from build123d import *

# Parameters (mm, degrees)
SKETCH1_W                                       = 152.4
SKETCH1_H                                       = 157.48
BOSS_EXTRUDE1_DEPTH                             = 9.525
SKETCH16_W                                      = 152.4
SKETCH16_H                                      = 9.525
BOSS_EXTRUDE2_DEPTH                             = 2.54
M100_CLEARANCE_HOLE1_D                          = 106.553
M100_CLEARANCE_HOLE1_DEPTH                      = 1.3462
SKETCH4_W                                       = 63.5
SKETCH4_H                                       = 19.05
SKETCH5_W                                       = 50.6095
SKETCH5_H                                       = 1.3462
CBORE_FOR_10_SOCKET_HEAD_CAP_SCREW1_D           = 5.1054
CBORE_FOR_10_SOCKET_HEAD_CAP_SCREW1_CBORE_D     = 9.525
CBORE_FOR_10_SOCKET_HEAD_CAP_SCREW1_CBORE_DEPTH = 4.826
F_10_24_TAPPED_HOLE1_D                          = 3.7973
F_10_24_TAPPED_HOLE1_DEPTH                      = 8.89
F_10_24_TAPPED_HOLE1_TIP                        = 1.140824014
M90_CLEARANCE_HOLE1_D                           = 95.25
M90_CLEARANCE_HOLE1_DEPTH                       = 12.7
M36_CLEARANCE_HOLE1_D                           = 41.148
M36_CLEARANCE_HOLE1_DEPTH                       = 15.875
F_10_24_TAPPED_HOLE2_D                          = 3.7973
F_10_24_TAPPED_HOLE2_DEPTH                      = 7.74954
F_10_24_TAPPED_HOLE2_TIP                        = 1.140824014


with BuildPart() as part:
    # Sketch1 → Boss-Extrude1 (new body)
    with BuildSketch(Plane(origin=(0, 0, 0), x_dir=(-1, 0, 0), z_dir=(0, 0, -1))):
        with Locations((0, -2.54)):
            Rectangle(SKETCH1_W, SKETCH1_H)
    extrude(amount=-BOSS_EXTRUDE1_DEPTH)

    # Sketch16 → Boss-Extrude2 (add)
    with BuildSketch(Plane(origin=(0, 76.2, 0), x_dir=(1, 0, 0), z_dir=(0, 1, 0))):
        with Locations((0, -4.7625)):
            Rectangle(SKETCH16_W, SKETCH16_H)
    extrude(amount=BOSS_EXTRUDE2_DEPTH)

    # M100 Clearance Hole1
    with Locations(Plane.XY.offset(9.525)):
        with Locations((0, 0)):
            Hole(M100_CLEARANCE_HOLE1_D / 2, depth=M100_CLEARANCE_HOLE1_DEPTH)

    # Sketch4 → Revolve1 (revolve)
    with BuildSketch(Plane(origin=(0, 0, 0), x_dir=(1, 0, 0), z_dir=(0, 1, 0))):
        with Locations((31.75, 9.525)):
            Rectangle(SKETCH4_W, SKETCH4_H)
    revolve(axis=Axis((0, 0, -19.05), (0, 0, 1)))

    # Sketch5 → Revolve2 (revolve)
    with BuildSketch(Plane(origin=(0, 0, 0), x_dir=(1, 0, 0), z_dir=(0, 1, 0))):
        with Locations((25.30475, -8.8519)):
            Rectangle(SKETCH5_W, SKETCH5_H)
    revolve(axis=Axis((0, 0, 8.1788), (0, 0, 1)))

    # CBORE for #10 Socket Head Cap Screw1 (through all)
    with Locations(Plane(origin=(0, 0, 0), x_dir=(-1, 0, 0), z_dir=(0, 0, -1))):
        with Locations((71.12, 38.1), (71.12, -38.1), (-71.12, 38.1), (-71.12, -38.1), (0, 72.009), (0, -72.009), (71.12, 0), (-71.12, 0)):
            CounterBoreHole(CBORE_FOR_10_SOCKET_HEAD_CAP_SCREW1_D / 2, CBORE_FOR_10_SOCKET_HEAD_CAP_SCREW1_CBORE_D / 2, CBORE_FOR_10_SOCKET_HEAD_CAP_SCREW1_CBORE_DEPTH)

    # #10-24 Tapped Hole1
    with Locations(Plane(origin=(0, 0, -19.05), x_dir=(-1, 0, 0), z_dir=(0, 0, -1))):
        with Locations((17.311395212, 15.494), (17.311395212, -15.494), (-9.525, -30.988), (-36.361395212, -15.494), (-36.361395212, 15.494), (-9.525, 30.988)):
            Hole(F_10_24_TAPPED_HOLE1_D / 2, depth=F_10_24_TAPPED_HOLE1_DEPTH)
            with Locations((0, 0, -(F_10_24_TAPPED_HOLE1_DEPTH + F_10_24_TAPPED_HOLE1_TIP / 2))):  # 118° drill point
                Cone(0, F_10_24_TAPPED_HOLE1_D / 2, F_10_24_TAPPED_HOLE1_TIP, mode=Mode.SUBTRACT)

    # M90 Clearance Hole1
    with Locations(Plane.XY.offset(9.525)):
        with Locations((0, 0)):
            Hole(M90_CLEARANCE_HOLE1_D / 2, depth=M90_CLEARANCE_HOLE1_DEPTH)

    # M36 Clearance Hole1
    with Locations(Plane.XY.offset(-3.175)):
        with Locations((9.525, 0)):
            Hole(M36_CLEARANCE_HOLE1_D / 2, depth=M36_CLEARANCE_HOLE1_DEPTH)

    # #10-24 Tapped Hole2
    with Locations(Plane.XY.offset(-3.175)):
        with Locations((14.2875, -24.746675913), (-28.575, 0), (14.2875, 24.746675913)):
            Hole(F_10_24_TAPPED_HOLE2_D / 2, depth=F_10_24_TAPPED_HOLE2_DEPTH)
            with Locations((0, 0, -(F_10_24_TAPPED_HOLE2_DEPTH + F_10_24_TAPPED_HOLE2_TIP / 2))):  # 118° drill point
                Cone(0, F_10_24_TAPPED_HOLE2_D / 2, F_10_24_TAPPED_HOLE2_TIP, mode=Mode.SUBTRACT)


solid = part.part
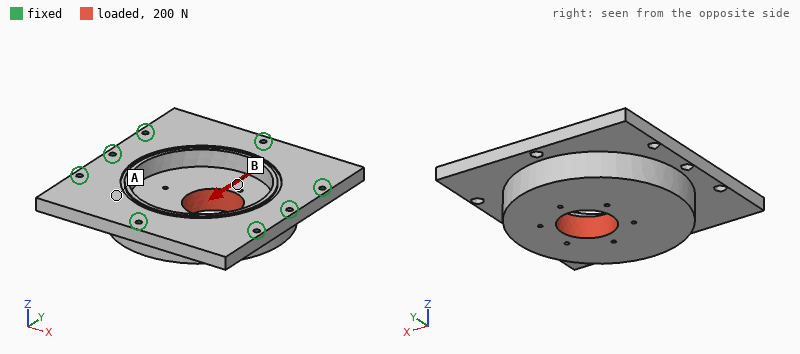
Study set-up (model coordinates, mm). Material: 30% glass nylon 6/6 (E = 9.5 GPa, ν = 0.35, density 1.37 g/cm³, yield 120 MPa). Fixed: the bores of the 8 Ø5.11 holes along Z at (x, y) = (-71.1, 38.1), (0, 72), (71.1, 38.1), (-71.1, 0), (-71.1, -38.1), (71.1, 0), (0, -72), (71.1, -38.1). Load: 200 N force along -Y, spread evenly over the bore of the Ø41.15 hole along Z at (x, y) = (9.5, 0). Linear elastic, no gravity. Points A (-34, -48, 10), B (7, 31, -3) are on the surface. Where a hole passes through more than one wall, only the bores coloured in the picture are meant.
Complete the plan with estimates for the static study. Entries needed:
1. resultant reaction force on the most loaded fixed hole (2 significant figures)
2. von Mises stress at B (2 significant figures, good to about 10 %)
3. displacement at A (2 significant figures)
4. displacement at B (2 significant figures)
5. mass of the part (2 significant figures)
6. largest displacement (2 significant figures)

43 N
0.12 MPa
0.45 µm
1.1 µm
490 g
1.4 µm
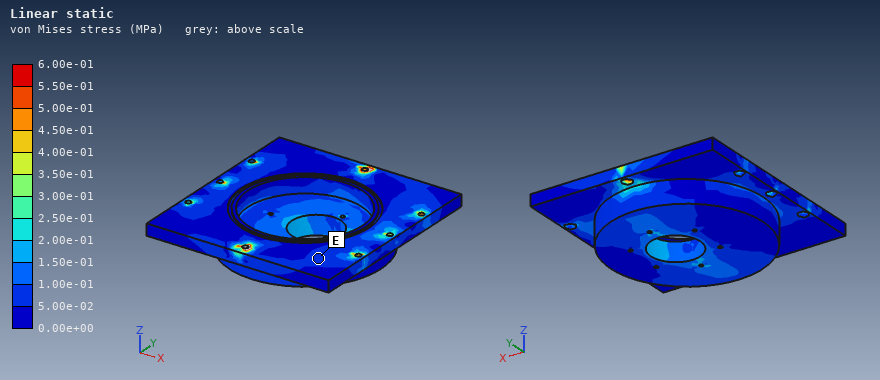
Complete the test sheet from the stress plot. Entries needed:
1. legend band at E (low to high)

5.00e-02 to 1.00e-01 MPa
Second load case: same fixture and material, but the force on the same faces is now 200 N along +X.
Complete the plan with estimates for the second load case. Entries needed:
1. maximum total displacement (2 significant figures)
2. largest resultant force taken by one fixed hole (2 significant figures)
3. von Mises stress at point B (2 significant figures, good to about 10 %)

1.5 µm
29 N
0.11 MPa
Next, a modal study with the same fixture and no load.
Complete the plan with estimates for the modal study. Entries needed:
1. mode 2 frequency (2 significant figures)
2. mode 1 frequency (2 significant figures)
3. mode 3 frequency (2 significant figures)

2500 Hz
2400 Hz
2500 Hz
